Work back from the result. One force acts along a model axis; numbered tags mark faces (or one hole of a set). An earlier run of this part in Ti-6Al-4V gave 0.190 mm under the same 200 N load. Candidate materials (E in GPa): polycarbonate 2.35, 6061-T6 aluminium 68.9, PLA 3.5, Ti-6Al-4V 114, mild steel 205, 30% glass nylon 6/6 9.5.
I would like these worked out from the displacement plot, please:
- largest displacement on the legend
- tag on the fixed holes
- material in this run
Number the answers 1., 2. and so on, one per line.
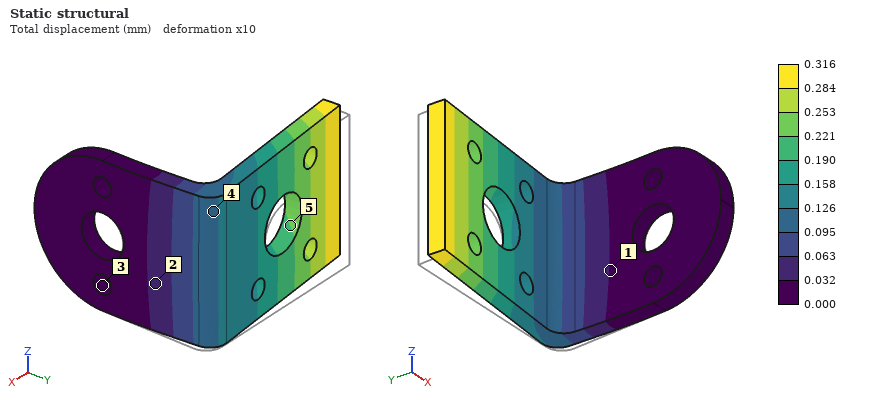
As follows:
1. 0.316 mm
2. 3
3. 6061-T6 aluminium
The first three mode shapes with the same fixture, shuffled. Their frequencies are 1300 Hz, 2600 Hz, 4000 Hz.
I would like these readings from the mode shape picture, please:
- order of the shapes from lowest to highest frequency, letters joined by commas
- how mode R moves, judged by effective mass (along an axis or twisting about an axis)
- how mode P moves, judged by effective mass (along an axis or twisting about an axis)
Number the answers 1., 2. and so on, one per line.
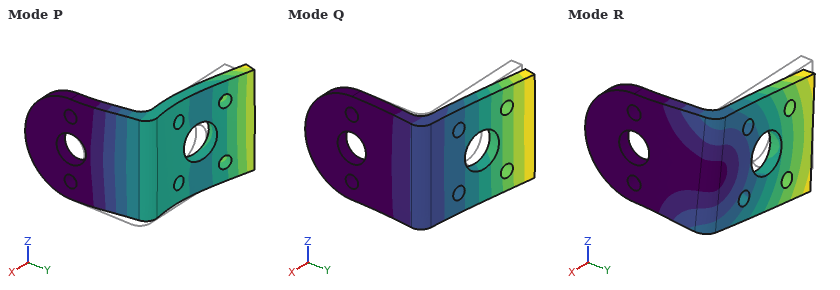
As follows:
1. Q, R, P
2. along Z
3. along X
